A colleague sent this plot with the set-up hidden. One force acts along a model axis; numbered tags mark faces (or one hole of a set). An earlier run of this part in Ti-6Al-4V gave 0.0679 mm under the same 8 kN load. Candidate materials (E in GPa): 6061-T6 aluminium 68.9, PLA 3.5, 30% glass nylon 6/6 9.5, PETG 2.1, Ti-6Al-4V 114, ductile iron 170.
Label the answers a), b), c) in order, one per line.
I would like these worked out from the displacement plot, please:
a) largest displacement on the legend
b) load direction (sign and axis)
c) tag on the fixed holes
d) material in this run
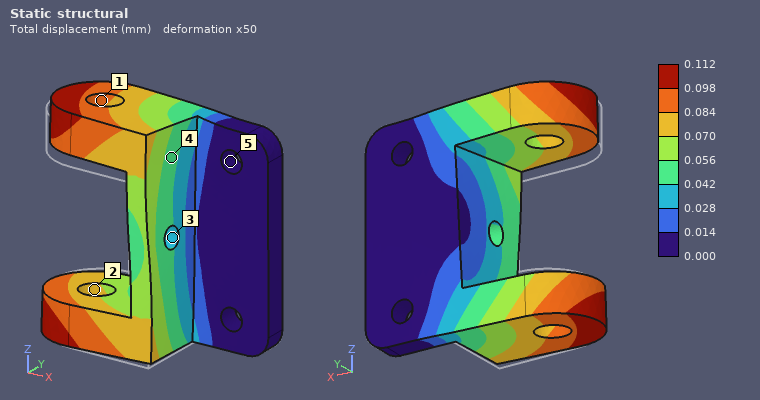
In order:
a) 0.112 mm
b) +Z
c) 5
d) 6061-T6 aluminium
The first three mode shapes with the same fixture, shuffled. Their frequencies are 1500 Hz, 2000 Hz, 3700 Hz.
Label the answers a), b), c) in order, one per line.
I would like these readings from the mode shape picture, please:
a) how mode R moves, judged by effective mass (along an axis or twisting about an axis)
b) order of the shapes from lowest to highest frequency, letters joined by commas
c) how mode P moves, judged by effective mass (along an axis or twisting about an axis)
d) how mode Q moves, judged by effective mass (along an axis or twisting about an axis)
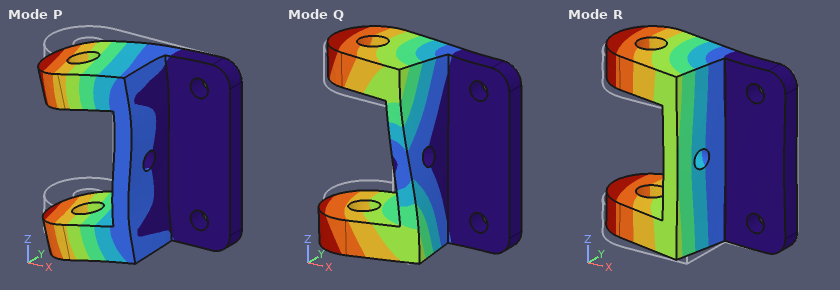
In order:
a) along Y
b) R, Q, P
c) along Z
d) twisting about X
